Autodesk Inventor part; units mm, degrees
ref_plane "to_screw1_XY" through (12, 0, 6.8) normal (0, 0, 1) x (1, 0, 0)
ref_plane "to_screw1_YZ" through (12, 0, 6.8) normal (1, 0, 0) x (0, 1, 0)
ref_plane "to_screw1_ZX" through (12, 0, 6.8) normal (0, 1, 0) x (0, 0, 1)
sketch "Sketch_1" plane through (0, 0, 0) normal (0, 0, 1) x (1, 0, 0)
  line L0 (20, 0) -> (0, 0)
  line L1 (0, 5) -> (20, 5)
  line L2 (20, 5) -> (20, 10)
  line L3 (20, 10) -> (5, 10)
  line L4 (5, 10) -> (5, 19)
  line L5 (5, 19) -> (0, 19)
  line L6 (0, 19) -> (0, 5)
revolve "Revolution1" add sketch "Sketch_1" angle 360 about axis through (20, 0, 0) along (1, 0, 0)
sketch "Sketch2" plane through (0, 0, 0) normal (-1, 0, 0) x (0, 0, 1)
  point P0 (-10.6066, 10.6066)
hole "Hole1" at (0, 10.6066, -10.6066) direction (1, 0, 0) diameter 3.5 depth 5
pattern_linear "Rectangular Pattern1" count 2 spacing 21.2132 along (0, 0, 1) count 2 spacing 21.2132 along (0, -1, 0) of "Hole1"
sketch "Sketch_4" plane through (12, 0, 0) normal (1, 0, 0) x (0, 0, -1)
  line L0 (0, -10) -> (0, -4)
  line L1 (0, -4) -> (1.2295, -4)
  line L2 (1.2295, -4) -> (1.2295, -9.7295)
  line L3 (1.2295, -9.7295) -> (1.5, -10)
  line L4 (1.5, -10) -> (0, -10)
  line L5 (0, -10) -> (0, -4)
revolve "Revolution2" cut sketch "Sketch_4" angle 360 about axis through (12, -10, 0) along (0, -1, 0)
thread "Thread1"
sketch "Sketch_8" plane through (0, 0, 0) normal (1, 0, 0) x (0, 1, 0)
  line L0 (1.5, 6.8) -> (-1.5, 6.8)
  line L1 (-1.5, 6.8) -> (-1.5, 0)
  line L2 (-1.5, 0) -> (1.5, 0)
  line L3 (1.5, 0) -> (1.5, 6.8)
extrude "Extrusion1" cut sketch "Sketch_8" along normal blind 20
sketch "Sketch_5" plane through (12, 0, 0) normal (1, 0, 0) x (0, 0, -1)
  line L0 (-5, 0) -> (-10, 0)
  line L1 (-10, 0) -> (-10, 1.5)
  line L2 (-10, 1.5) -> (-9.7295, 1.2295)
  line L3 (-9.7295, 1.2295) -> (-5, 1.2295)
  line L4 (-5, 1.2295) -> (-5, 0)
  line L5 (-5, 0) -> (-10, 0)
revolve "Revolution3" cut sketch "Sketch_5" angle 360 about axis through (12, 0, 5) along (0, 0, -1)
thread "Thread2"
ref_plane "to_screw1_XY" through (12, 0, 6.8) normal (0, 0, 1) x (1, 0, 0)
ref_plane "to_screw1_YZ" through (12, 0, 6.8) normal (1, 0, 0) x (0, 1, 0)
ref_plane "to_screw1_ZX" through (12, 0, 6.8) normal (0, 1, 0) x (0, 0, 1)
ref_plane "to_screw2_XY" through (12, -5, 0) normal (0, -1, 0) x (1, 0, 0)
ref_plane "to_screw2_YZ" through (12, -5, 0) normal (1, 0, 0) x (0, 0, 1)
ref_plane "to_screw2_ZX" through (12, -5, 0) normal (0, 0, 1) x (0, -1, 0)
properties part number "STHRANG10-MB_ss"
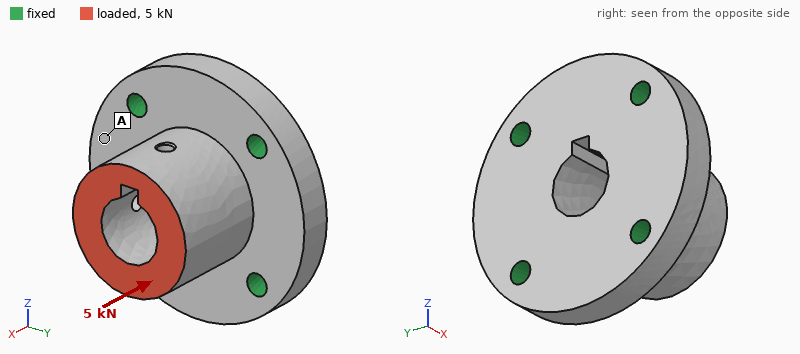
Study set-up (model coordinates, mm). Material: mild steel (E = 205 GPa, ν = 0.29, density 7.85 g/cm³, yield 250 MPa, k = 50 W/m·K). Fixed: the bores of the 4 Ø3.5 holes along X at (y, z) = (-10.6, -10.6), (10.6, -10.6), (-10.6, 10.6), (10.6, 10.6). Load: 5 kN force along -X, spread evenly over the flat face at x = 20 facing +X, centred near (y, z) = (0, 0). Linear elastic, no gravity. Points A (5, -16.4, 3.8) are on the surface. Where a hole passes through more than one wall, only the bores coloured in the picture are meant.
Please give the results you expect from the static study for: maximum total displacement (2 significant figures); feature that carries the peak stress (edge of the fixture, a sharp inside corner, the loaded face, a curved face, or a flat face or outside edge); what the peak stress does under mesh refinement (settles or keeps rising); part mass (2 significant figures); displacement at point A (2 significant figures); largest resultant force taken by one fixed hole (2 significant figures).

5.1 µm
edge of the fixture
keeps rising
66 g
0.87 µm
1.3 kN
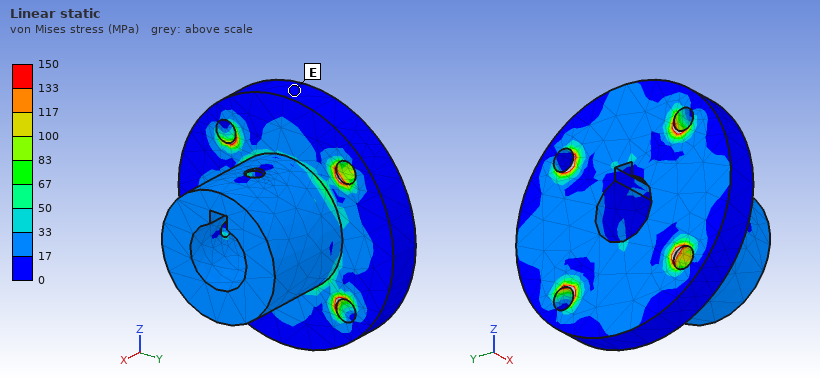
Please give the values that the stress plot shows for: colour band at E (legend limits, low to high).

0 to 17 MPa
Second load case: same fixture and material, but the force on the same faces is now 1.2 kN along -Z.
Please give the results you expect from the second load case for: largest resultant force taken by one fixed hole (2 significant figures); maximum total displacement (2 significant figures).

630 N
6.6 µm
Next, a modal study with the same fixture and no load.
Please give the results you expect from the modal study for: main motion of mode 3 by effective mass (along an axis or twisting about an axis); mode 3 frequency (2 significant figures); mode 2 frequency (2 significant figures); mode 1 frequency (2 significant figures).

along X
29 kHz
21 kHz
21 kHz
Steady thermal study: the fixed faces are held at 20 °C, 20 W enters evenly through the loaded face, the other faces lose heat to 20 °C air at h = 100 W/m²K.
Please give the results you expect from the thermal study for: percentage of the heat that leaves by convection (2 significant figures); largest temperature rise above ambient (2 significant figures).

21 %
34 K
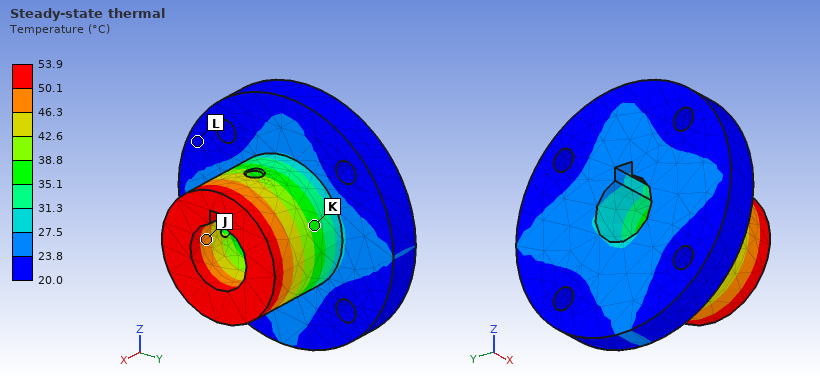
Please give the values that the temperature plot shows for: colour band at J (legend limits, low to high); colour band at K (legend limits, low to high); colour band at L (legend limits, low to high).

46.3 to 50.1 °C
35.1 to 38.8 °C
20.0 to 23.8 °C
